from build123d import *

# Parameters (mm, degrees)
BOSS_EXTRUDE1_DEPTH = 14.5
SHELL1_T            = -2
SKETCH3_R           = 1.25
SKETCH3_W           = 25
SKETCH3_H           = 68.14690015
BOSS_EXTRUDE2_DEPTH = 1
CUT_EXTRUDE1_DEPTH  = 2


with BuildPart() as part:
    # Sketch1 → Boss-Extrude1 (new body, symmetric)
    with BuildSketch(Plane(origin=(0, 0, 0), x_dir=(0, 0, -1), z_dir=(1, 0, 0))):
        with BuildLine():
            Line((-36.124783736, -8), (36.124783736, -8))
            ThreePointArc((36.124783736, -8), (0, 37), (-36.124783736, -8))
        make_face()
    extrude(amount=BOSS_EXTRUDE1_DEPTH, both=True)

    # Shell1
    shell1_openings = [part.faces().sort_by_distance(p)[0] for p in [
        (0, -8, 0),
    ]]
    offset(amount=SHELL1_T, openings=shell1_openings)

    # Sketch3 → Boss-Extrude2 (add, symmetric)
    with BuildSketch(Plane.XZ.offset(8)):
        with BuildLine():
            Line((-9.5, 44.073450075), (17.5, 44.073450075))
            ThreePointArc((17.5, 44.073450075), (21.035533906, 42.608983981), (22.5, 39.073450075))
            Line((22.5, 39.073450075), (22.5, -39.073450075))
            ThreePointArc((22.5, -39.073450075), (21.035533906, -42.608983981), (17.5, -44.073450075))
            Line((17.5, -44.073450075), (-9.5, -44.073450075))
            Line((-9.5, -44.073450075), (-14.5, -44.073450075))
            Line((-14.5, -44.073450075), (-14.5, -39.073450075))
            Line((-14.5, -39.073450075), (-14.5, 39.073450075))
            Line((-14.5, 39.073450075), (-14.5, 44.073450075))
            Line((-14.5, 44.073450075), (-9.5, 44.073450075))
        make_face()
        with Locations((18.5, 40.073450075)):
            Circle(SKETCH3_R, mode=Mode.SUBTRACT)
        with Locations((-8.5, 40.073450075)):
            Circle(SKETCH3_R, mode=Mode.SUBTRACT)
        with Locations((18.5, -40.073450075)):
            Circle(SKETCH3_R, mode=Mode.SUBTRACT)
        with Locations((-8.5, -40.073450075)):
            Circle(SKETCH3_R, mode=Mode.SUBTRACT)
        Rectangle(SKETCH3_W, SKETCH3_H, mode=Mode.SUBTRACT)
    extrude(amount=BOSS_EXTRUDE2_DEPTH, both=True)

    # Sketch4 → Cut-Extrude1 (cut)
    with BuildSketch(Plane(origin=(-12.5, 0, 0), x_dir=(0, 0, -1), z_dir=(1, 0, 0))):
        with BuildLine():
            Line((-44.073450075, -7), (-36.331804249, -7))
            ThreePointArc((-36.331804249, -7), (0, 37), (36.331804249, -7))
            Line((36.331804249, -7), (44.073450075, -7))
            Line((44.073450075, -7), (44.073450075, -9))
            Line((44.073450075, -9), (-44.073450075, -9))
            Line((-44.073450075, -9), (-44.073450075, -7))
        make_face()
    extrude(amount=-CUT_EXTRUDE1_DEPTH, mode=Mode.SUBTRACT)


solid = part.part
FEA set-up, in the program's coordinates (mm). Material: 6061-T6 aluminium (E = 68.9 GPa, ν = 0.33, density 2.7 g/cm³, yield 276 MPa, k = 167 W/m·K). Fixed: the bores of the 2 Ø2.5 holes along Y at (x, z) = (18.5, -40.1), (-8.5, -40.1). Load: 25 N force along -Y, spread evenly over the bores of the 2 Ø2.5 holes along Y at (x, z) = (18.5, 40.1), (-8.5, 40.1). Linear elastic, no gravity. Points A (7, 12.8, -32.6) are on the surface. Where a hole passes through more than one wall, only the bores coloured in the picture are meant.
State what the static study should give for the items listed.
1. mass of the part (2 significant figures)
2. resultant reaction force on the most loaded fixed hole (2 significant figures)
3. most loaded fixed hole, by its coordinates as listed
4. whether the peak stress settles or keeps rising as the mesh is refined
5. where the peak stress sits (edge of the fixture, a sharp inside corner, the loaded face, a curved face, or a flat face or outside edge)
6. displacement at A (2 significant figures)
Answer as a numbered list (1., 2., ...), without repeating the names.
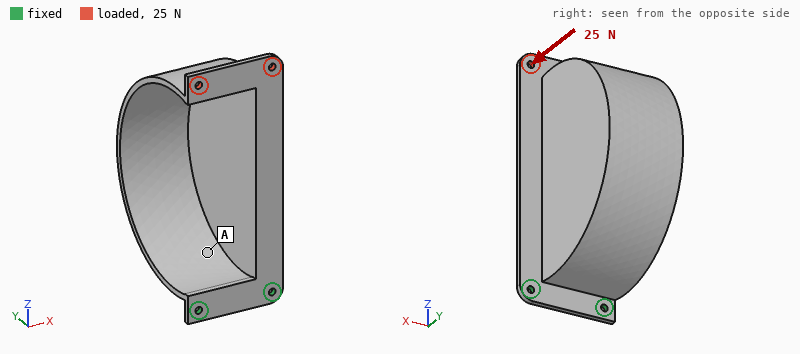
1. 39 g
2. 15 N
3. (18.5, -40.1)
4. keeps rising
5. edge of the fixture
6. 0.25 mm
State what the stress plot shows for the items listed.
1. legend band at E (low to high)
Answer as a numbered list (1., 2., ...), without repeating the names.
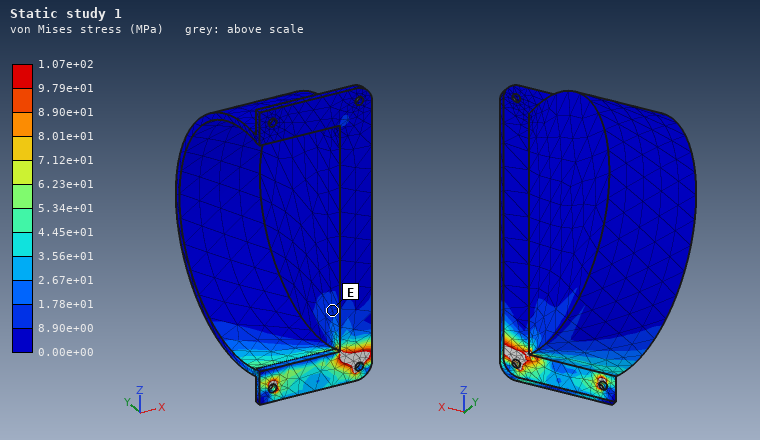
1. 8.90e+00 to 1.78e+01 MPa
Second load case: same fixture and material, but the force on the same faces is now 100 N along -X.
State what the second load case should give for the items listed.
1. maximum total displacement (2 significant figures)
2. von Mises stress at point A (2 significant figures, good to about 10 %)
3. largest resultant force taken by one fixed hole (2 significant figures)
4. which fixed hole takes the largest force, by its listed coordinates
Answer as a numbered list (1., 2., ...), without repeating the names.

1. 1.1 mm
2. 25 MPa
3. 360 N
4. (-8.5, -40.1)
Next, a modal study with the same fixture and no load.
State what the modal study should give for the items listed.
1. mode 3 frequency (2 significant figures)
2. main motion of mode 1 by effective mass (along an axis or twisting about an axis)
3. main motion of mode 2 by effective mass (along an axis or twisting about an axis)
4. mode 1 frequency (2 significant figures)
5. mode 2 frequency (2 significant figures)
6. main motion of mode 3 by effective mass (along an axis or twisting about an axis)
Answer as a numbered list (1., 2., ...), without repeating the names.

1. 1200 Hz
2. along Y
3. along X
4. 190 Hz
5. 500 Hz
6. twisting about Z
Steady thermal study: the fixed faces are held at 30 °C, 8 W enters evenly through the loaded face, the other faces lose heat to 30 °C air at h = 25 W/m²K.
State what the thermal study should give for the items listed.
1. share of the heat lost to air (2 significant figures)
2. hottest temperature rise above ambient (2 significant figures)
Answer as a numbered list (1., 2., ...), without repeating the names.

1. 59 %
2. 36 K
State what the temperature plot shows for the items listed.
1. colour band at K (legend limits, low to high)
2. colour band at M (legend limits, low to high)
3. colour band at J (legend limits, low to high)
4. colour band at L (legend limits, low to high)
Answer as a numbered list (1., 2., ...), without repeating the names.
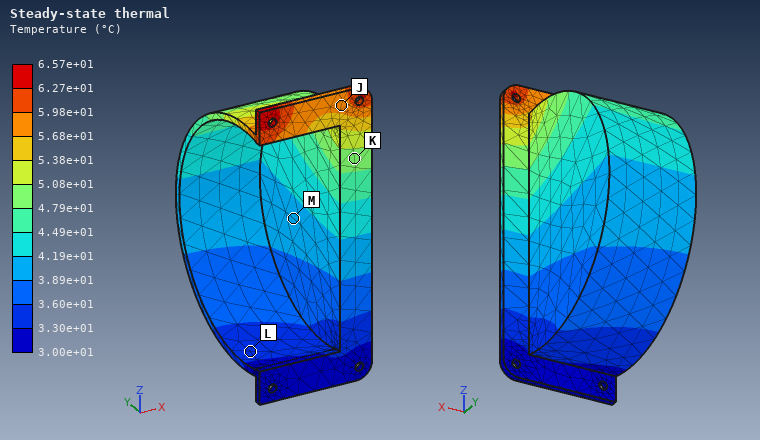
1. 4.79e+01 to 5.08e+01 °C
2. 3.89e+01 to 4.19e+01 °C
3. 5.68e+01 to 5.98e+01 °C
4. 3.30e+01 to 3.60e+01 °C
